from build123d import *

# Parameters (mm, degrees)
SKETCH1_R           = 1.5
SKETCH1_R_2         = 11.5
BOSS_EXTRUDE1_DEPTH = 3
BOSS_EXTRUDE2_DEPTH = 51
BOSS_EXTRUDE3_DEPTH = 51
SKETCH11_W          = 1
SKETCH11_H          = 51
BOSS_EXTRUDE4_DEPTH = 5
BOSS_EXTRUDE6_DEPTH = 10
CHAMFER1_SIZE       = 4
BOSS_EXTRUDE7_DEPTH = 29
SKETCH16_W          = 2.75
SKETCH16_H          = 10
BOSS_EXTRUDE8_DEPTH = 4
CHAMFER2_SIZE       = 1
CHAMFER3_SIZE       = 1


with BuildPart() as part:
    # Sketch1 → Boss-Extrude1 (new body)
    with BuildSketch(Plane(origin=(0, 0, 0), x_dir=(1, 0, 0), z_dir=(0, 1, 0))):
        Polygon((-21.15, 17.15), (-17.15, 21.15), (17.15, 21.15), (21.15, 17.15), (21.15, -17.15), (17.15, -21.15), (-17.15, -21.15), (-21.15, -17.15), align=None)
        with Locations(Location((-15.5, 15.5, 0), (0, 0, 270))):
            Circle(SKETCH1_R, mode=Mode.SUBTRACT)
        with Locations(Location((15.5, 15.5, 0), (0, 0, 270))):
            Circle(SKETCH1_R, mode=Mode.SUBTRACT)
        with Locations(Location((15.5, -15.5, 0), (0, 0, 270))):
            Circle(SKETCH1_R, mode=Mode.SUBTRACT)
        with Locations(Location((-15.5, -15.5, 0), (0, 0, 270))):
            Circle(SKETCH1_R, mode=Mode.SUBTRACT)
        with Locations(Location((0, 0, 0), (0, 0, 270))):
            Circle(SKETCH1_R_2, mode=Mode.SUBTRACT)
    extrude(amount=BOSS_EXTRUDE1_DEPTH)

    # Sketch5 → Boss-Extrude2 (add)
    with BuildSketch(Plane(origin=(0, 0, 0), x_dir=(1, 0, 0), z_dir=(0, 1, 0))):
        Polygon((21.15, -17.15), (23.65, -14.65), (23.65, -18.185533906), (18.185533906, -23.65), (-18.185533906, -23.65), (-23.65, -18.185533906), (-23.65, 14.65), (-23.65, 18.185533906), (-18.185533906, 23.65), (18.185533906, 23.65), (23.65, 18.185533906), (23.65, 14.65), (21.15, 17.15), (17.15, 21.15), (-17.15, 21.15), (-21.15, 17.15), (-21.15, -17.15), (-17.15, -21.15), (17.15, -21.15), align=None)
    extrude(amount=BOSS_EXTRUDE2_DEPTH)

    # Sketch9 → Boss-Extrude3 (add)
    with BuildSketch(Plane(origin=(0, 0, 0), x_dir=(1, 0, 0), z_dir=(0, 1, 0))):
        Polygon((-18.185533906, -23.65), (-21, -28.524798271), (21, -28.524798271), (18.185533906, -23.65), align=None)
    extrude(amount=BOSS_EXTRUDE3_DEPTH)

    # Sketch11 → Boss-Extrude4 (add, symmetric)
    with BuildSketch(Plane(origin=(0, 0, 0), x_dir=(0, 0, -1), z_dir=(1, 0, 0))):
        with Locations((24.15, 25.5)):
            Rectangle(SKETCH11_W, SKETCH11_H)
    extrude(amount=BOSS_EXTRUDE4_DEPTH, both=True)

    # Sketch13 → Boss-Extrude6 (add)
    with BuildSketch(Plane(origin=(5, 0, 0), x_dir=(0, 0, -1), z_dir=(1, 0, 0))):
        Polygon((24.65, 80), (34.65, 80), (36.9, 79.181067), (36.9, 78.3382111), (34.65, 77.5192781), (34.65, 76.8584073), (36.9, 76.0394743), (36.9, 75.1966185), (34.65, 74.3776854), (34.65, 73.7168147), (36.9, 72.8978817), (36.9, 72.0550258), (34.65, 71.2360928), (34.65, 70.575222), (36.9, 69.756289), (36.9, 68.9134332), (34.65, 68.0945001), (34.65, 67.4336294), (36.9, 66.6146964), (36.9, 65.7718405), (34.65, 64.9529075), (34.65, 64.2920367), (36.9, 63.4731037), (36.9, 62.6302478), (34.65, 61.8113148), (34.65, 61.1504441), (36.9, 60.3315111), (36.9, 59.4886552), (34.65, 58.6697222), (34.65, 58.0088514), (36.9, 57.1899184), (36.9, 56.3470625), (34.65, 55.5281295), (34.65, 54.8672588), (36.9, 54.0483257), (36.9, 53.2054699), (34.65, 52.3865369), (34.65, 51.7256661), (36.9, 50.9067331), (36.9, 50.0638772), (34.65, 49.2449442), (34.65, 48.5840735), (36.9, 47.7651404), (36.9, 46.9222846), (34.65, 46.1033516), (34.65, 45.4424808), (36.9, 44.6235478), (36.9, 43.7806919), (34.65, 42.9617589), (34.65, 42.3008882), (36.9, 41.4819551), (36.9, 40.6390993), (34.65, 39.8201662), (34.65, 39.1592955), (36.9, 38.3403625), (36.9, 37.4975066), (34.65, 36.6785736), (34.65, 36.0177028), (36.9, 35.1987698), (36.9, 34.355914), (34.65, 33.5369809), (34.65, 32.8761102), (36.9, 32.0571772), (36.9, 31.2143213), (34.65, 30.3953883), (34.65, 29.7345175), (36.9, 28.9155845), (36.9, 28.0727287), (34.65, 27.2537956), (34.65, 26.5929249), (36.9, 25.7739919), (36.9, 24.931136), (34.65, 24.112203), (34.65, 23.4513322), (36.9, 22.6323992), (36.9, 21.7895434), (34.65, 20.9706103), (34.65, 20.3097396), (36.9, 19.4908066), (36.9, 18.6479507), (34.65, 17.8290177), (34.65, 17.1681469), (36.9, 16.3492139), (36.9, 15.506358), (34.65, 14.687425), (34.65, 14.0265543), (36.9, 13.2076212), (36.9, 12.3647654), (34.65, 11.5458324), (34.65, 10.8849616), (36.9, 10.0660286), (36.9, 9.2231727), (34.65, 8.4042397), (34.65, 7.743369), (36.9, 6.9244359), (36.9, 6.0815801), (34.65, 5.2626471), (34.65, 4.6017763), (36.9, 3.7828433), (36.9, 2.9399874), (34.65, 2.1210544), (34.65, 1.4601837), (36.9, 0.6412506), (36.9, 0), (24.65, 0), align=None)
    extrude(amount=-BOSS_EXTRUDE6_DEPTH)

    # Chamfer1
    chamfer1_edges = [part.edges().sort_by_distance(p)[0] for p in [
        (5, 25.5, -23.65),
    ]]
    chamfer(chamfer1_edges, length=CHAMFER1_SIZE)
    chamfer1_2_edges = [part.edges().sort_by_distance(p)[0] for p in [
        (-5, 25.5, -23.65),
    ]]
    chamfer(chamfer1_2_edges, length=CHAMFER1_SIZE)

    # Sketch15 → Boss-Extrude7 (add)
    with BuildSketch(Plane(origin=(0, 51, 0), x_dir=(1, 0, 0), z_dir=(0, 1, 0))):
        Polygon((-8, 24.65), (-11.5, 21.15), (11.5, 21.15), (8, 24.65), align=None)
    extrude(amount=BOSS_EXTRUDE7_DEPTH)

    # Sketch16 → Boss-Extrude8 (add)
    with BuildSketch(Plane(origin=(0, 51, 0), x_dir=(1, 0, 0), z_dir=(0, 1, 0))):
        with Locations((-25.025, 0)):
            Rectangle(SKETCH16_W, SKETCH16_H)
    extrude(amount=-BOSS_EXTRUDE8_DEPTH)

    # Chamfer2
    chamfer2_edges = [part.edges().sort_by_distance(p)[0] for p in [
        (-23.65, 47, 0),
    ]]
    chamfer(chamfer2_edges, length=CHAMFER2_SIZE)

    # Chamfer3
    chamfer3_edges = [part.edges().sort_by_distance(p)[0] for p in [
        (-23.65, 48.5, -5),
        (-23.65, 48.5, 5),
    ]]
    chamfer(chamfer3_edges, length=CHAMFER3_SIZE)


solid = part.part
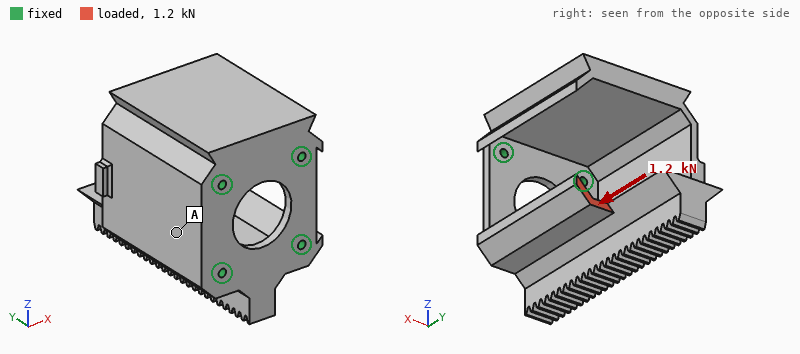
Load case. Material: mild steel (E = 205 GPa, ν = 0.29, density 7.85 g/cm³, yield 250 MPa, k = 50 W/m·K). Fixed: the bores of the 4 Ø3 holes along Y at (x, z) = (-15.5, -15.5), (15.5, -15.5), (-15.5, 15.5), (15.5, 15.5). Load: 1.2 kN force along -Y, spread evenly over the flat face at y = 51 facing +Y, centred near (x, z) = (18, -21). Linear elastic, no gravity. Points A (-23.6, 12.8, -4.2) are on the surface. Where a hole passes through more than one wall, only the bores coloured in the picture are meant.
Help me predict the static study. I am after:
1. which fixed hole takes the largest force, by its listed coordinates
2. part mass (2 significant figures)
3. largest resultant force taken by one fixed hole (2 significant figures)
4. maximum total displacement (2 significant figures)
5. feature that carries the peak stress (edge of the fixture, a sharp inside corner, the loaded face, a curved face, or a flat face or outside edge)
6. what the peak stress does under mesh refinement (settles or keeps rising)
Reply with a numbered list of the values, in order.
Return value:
1. (15.5, -15.5)
2. 340 g
3. 1.2 kN
4. 32 µm
5. edge of the fixture
6. keeps rising
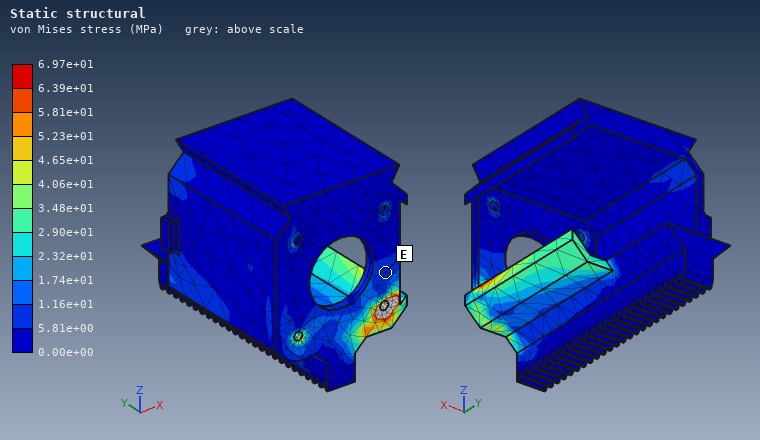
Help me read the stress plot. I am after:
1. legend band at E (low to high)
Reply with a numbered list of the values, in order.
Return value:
1. 5.81e+00 to 1.16e+01 MPa
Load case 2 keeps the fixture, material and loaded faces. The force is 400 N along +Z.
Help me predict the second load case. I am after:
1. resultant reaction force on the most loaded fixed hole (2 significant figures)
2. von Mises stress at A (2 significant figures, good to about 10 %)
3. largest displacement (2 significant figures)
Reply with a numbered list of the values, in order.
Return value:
1. 680 N
2. 13 MPa
3. 0.20 mm
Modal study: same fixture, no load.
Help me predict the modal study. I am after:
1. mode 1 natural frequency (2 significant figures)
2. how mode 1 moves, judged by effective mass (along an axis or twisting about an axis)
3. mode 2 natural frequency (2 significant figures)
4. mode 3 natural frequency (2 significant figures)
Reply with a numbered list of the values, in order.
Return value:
1. 1100 Hz
2. along Z
3. 2000 Hz
4. 2700 Hz
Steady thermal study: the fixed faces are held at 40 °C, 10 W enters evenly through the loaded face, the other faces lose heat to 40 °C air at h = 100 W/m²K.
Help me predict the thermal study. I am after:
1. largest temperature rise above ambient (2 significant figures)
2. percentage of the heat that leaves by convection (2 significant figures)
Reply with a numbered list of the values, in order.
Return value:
1. 68 K
2. 85 %
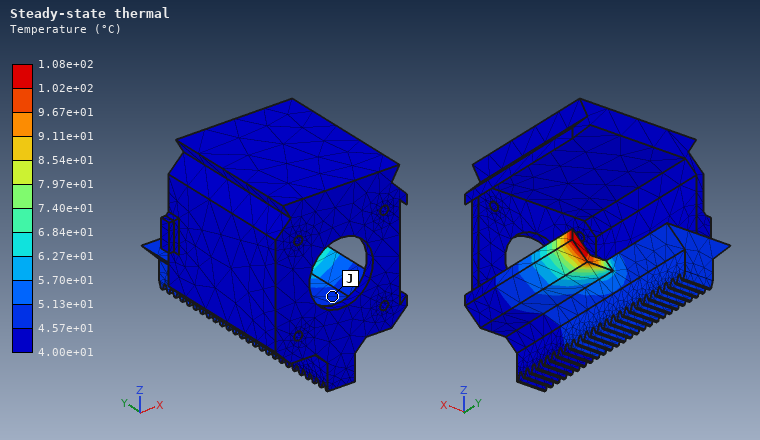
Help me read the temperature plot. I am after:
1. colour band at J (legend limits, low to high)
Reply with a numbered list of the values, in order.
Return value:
1. 4.57e+01 to 5.13e+01 °C
